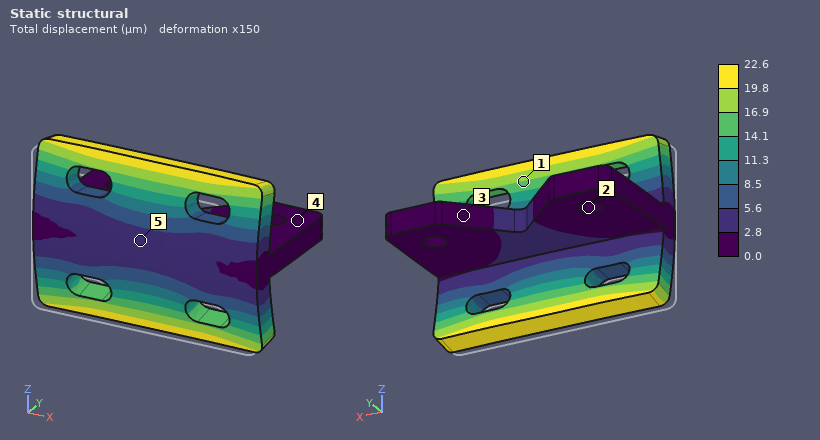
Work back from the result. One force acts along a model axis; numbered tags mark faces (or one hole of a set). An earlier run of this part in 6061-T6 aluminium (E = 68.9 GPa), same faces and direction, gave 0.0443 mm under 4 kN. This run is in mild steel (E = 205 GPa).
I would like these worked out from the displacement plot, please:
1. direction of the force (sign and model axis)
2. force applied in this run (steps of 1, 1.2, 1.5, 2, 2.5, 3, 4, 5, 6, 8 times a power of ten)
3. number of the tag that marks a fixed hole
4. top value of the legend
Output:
+Y
6 kN
2
22.6 µm
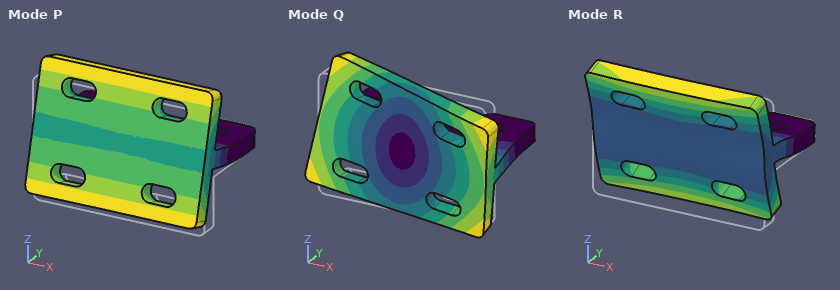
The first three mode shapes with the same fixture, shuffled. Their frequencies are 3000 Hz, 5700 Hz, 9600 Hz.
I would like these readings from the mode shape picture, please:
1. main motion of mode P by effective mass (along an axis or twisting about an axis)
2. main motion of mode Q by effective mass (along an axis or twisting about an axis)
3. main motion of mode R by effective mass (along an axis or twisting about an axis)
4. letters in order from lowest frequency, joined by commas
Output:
along Z
twisting about Y
along Z
P, Q, R
